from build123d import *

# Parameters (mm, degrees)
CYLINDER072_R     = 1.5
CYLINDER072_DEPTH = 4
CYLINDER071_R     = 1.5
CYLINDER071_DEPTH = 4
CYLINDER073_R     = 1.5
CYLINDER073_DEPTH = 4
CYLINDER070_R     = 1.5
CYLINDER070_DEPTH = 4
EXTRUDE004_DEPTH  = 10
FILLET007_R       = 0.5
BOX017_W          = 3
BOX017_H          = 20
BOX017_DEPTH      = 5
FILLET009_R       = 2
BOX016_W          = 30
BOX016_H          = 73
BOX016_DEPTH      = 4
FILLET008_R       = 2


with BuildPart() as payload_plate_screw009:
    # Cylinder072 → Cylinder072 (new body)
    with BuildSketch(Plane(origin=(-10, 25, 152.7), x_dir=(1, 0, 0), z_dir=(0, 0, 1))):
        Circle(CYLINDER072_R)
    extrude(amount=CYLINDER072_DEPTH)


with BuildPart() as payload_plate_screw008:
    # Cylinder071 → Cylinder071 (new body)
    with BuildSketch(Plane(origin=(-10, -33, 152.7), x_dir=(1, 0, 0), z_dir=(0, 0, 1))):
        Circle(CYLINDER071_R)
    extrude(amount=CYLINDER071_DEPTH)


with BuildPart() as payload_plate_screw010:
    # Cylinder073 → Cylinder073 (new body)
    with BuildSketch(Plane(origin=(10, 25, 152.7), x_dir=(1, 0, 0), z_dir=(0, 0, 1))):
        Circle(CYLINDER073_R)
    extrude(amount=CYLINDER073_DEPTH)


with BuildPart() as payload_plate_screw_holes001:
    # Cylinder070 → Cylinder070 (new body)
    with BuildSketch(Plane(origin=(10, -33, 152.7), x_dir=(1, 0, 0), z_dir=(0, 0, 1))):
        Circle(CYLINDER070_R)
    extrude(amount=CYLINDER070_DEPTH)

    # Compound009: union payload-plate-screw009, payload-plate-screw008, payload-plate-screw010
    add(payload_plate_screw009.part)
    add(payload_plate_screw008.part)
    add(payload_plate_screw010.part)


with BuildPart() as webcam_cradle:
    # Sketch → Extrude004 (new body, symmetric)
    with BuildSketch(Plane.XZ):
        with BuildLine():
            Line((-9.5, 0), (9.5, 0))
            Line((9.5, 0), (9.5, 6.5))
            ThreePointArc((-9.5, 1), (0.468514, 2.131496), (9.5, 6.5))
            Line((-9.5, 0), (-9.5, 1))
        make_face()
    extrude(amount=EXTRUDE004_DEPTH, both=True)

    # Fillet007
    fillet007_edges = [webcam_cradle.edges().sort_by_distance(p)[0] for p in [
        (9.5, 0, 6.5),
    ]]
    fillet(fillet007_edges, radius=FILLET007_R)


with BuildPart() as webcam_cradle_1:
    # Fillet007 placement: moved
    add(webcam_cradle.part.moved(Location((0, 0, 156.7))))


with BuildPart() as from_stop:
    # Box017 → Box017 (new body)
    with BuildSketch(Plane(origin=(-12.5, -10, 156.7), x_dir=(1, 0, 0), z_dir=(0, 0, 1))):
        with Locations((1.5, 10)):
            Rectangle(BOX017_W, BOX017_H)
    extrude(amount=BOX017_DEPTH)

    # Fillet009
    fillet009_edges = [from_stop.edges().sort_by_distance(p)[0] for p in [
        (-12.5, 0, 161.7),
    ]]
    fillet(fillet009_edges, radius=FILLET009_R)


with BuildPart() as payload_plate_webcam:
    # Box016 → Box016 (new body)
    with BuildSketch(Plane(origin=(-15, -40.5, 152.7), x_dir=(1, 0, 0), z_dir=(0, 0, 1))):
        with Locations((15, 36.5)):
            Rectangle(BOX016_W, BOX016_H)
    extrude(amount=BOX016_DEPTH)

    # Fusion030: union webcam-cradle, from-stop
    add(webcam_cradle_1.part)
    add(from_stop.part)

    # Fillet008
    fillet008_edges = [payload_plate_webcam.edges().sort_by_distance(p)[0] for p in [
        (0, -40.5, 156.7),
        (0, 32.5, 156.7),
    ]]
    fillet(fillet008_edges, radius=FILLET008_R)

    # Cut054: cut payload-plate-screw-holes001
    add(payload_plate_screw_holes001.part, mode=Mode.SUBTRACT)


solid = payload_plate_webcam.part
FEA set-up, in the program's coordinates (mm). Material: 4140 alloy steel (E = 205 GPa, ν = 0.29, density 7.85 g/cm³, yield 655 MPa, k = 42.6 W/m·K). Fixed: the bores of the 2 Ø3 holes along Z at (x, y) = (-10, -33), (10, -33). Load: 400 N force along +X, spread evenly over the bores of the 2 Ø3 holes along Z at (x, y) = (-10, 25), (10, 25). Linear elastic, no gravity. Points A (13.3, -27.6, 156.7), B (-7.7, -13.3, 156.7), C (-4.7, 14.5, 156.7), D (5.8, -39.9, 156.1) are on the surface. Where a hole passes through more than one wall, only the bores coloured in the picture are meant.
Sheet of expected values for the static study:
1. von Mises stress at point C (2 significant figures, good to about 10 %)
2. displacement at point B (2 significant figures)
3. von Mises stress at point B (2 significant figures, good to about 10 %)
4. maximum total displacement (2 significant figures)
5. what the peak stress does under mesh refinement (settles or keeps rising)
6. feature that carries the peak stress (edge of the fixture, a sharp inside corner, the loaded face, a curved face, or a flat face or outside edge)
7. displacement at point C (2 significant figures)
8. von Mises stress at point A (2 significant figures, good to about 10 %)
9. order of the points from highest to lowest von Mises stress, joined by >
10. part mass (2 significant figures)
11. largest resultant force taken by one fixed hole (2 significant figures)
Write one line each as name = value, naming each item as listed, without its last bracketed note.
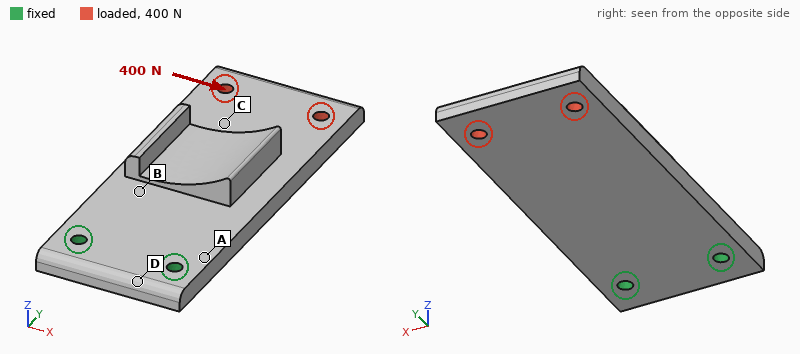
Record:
von Mises stress at point C = 8.3 MPa
displacement at point B = 3.8 µm
von Mises stress at point B = 16 MPa
maximum total displacement = 21 µm
what the peak stress does under mesh refinement = keeps rising
feature that carries the peak stress = edge of the fixture
displacement at point C = 13 µm
von Mises stress at point A = 29 MPa
order of the points from highest to lowest von Mises stress, joined by > = A > B > C > D
part mass = 77 g
largest resultant force taken by one fixed hole = 1.1 kN
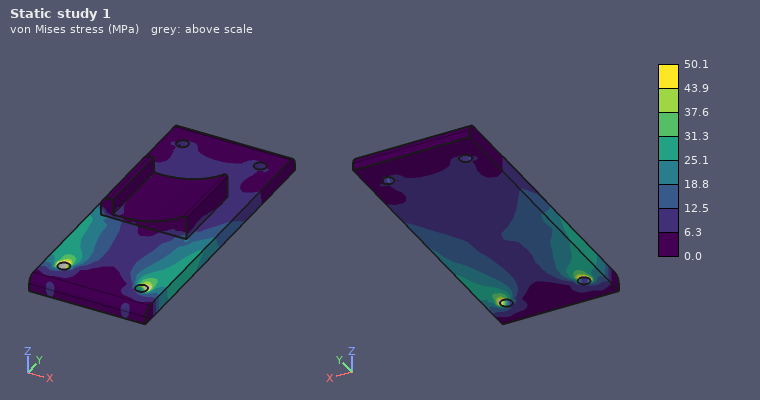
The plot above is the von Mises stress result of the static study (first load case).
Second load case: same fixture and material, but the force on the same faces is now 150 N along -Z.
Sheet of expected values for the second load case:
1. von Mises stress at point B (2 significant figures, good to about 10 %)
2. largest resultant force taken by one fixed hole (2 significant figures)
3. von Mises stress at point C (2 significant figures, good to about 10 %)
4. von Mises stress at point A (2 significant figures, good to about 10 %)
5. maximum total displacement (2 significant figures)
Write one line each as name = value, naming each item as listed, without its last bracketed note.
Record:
von Mises stress at point B = 68 MPa
largest resultant force taken by one fixed hole = 76 N
von Mises stress at point C = 18 MPa
von Mises stress at point A = 100 MPa
maximum total displacement = 0.31 mm
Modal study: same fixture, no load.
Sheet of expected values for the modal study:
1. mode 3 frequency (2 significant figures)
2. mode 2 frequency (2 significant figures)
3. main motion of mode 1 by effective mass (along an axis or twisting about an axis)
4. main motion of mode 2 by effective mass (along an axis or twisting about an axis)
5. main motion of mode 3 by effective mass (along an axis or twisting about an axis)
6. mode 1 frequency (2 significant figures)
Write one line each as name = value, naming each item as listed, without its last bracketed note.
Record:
mode 3 frequency = 4800 Hz
mode 2 frequency = 3900 Hz
main motion of mode 1 by effective mass = along Z
main motion of mode 2 by effective mass = twisting about Y
main motion of mode 3 by effective mass = along X
mode 1 frequency = 770 Hz
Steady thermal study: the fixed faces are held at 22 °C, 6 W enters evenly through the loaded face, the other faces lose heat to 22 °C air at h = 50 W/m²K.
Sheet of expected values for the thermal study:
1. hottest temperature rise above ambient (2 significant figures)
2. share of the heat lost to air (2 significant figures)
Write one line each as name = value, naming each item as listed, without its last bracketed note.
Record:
hottest temperature rise above ambient = 36 K
share of the heat lost to air = 66 %
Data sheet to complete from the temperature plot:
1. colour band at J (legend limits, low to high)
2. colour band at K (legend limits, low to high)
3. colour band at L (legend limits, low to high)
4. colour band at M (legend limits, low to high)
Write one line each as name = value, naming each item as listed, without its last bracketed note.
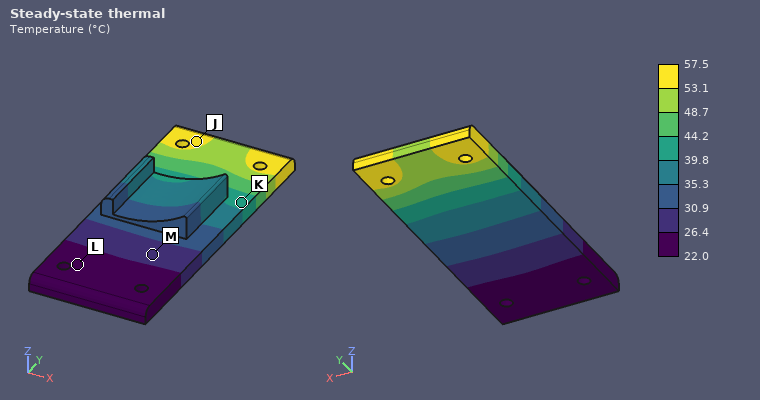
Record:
colour band at J = 53.1 to 57.5 °C
colour band at K = 39.8 to 44.2 °C
colour band at L = 22.0 to 26.4 °C
colour band at M = 26.4 to 30.9 °C
